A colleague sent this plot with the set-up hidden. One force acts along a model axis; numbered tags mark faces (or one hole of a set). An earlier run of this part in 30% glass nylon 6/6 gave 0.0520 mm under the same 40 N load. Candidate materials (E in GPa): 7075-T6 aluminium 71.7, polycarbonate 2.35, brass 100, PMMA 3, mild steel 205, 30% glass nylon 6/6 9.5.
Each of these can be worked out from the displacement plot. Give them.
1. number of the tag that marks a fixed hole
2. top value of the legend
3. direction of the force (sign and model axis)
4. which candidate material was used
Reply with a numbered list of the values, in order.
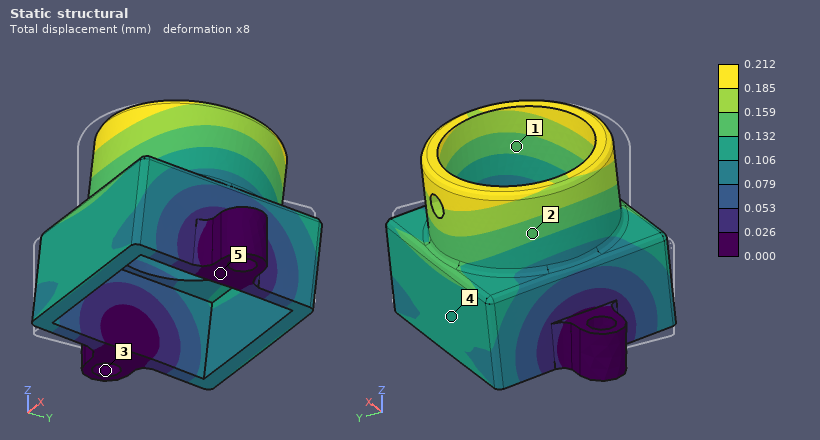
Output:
1. 3
2. 0.212 mm
3. +Y
4. polycarbonate
